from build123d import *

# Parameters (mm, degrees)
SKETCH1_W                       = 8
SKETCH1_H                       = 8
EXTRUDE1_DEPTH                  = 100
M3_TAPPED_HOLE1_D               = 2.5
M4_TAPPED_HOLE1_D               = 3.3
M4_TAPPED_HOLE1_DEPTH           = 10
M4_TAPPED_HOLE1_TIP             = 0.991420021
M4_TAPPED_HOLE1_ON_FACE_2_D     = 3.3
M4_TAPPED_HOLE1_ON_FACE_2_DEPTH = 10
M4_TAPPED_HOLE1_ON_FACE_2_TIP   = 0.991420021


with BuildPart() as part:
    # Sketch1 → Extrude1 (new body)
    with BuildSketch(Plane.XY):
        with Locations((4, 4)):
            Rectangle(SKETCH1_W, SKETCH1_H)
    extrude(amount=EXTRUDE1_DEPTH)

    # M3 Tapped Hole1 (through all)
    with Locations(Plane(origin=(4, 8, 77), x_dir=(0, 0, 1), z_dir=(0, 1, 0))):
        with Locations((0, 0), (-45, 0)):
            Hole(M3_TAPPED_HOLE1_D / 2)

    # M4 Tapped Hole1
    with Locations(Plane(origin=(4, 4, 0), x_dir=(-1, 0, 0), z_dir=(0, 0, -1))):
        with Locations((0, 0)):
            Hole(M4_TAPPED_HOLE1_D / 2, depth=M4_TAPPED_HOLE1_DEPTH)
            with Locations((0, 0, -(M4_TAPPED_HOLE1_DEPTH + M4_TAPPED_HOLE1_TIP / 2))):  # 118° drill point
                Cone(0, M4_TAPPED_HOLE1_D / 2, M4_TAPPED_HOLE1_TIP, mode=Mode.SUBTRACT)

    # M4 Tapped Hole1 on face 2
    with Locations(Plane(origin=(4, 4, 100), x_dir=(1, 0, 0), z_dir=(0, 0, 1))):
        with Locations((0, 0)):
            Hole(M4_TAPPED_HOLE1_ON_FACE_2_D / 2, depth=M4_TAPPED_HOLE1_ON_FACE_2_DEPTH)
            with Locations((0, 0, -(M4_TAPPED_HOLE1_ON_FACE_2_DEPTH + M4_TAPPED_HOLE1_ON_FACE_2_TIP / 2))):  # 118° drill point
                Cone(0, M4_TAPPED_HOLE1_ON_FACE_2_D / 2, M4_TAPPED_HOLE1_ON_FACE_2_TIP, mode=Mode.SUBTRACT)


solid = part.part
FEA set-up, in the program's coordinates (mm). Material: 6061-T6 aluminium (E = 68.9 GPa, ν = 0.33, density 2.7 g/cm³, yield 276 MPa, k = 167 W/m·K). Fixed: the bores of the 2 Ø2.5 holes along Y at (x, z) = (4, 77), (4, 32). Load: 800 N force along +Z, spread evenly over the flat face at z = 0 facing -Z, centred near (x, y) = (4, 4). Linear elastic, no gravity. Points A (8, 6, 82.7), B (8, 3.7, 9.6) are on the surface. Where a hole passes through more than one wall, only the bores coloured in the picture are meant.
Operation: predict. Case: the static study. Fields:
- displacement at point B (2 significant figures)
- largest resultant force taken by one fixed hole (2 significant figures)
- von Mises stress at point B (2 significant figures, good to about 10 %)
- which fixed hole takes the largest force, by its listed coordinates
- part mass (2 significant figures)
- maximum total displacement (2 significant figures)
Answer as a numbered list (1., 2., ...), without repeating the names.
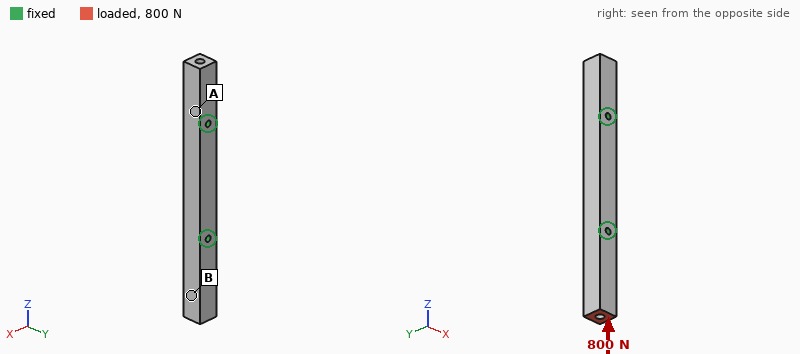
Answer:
1. 4.2 µm
2. 780 N
3. 14 MPa
4. (4, 32)
5. 17 g
6. 6.2 µm
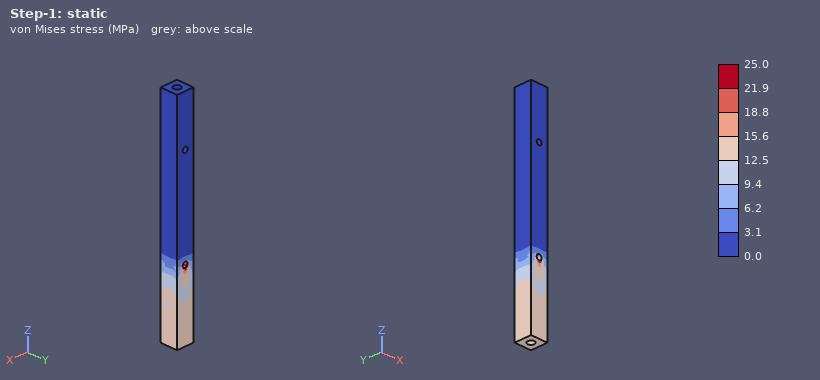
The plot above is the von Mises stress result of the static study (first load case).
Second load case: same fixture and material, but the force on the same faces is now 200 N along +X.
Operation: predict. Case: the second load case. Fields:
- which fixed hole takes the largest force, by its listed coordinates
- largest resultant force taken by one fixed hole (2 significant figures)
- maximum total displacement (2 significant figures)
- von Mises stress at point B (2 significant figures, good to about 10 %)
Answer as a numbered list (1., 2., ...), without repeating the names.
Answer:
1. (4, 32)
2. 250 N
3. 0.13 mm
4. 23 MPa
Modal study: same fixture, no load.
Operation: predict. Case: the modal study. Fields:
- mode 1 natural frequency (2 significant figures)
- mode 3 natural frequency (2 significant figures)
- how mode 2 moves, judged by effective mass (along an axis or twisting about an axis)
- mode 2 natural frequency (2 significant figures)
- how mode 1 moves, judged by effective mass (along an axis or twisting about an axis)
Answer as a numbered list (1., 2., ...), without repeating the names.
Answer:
1. 5500 Hz
2. 9700 Hz
3. along Y
4. 6400 Hz
5. along X
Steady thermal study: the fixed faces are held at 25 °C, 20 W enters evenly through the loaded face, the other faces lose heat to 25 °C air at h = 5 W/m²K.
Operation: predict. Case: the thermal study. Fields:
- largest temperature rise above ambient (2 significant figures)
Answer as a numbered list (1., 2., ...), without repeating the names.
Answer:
1. 62 K
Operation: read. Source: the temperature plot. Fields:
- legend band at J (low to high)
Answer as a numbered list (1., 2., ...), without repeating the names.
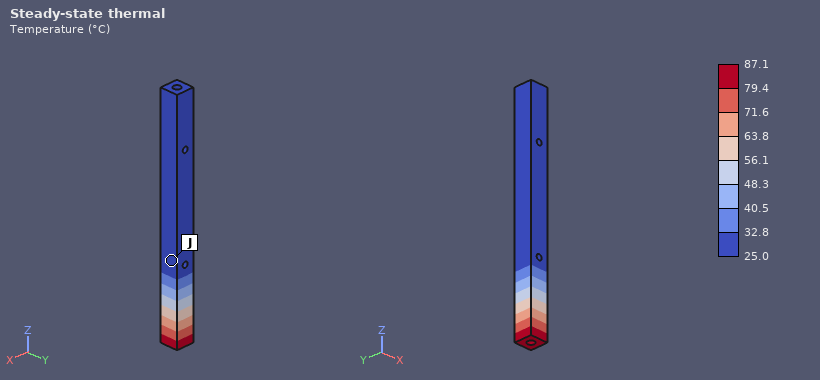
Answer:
1. 25.0 to 32.8 °C
